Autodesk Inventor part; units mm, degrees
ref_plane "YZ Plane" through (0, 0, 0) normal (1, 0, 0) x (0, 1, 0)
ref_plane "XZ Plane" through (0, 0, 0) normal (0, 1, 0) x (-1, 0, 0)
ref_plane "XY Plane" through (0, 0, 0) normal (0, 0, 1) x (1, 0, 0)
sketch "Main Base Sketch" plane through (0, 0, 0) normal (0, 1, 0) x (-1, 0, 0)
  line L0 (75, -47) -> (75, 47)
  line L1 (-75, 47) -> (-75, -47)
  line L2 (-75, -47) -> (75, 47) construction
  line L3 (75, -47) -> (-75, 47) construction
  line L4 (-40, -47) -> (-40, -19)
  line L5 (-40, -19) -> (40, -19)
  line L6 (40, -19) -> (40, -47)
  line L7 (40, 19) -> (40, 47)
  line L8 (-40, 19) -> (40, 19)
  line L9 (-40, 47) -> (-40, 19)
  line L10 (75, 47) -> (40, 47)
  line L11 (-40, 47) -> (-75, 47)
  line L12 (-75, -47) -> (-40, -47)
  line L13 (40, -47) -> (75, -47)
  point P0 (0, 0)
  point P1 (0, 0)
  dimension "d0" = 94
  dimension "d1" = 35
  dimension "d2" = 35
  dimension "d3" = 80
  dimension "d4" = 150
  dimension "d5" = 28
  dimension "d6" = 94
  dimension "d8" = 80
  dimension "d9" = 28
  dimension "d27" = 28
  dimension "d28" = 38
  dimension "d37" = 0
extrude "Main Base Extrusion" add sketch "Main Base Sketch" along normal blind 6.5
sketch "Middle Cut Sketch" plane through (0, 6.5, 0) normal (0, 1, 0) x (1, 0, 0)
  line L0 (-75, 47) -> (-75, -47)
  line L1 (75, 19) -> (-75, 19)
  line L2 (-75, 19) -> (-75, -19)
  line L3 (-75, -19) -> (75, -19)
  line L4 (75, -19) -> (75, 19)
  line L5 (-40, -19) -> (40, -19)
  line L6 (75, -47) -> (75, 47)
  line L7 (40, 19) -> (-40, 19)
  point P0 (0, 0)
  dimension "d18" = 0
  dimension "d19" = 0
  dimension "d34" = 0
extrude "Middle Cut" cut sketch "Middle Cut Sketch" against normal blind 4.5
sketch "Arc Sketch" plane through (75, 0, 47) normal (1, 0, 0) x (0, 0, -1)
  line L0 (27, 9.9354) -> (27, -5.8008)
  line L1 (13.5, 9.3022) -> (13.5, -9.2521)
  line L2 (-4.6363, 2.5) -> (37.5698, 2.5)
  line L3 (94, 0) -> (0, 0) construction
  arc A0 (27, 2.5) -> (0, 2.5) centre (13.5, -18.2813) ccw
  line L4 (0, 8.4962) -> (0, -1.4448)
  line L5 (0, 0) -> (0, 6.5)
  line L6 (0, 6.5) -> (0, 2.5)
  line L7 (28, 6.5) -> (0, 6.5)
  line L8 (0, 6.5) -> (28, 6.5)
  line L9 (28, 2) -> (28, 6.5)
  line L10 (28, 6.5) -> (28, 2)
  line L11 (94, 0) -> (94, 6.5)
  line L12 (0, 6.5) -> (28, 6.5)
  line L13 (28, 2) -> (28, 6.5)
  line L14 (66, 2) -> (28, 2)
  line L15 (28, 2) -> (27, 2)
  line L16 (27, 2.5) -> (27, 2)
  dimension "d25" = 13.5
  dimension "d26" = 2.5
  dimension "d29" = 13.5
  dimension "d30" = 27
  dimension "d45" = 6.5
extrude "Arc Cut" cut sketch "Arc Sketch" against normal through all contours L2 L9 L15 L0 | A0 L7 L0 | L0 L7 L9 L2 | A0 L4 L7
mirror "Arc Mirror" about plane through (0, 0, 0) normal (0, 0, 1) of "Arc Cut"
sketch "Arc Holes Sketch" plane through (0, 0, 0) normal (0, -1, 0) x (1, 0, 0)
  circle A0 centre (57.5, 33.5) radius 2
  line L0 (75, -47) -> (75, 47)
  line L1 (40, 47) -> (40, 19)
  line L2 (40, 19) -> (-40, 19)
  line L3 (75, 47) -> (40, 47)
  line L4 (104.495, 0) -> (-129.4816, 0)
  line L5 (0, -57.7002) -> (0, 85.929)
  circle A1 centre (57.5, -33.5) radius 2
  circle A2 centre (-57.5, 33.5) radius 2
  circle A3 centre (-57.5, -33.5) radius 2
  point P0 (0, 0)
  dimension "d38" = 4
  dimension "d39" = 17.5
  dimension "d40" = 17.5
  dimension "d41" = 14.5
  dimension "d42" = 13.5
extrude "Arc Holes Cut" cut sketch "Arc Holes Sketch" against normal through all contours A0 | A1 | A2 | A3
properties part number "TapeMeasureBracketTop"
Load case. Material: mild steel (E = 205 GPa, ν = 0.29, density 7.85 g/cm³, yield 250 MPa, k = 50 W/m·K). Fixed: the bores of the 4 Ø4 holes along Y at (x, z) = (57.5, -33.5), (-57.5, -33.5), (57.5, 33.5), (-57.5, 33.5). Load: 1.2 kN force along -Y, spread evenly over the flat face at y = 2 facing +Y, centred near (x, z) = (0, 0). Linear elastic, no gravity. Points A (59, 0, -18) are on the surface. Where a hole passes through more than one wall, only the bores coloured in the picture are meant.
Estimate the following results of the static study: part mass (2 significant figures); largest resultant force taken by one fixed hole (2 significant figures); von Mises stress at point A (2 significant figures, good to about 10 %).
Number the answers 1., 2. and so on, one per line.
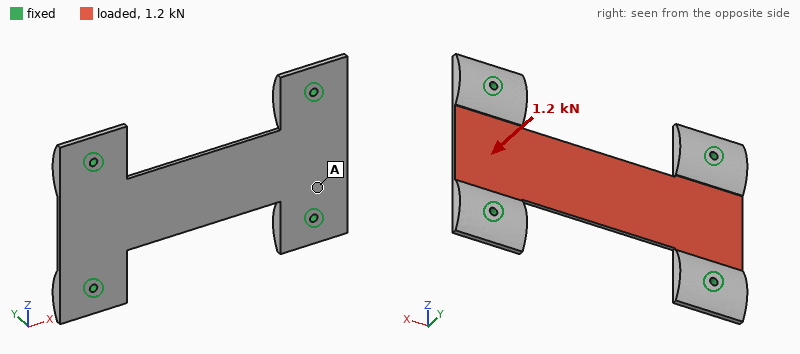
1. 240 g
2. 620 N
3. 25 MPa
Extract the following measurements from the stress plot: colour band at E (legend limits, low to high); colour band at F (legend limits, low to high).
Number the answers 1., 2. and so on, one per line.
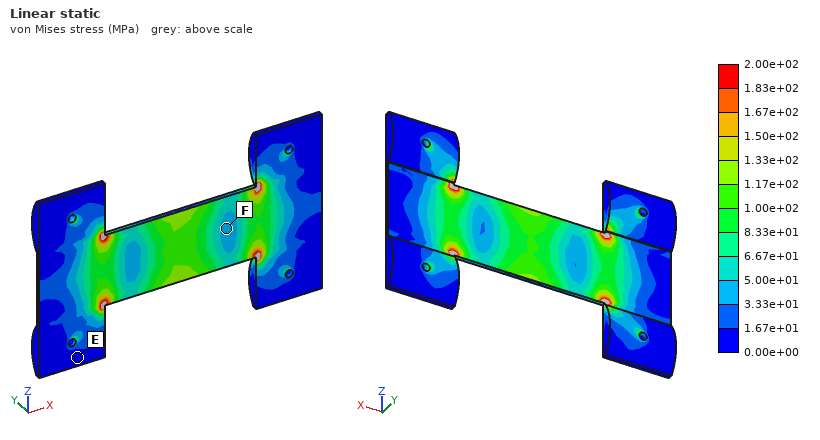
1. 0.00e+00 to 1.67e+01 MPa
2. 3.33e+01 to 5.00e+01 MPa
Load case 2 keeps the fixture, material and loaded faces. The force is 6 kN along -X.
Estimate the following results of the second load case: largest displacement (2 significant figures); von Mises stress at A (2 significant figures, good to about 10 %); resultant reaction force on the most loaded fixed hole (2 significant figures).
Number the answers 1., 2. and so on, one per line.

1. 14 µm
2. 38 MPa
3. 1.5 kN
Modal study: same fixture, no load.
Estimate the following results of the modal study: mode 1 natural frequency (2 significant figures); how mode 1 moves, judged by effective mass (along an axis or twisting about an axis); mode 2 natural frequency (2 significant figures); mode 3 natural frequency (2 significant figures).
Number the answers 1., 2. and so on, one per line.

1. 1100 Hz
2. along Y
3. 2400 Hz
4. 2900 Hz
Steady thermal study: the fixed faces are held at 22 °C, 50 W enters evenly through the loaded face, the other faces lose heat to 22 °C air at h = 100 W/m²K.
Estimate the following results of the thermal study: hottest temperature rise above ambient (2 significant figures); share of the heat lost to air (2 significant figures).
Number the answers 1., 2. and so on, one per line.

1. 57 K
2. 57 %
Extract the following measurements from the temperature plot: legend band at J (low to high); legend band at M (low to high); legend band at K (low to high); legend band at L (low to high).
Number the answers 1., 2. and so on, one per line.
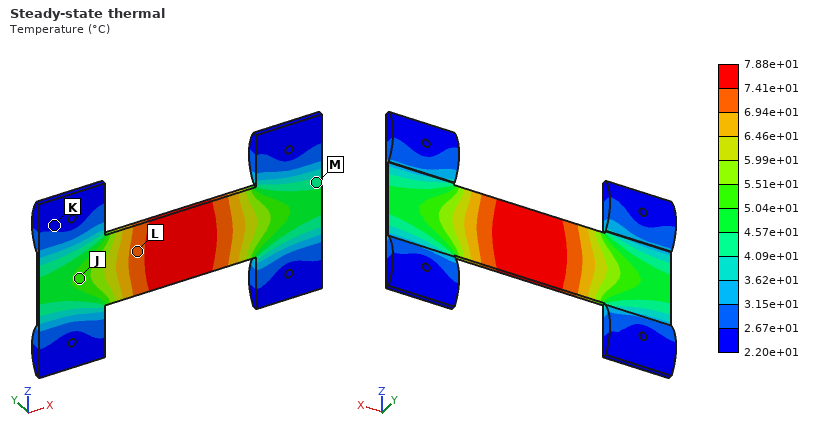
1. 5.04e+01 to 5.51e+01 °C
2. 4.09e+01 to 4.57e+01 °C
3. 2.20e+01 to 2.67e+01 °C
4. 6.94e+01 to 7.41e+01 °C
